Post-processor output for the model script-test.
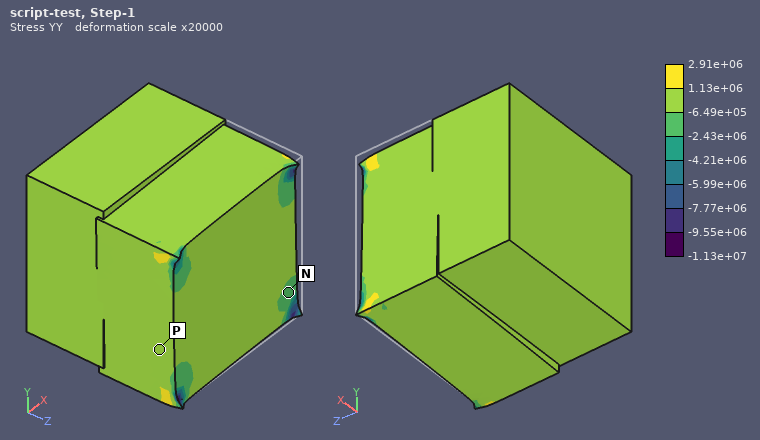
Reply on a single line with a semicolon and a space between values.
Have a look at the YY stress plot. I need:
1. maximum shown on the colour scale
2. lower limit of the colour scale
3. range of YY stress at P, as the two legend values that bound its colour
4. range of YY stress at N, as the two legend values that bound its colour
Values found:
2.91e+06; -1.13e+07; -6.49e+05 to 1.13e+06; -2.43e+06 to -6.49e+05
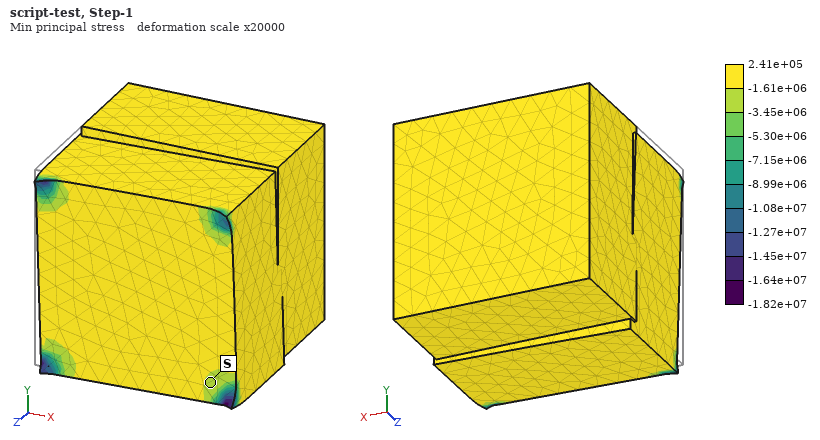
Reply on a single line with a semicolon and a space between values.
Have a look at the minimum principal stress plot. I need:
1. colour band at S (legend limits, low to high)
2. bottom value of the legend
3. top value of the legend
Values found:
-3.45e+06 to -1.61e+06; -1.82e+07; 2.41e+05
